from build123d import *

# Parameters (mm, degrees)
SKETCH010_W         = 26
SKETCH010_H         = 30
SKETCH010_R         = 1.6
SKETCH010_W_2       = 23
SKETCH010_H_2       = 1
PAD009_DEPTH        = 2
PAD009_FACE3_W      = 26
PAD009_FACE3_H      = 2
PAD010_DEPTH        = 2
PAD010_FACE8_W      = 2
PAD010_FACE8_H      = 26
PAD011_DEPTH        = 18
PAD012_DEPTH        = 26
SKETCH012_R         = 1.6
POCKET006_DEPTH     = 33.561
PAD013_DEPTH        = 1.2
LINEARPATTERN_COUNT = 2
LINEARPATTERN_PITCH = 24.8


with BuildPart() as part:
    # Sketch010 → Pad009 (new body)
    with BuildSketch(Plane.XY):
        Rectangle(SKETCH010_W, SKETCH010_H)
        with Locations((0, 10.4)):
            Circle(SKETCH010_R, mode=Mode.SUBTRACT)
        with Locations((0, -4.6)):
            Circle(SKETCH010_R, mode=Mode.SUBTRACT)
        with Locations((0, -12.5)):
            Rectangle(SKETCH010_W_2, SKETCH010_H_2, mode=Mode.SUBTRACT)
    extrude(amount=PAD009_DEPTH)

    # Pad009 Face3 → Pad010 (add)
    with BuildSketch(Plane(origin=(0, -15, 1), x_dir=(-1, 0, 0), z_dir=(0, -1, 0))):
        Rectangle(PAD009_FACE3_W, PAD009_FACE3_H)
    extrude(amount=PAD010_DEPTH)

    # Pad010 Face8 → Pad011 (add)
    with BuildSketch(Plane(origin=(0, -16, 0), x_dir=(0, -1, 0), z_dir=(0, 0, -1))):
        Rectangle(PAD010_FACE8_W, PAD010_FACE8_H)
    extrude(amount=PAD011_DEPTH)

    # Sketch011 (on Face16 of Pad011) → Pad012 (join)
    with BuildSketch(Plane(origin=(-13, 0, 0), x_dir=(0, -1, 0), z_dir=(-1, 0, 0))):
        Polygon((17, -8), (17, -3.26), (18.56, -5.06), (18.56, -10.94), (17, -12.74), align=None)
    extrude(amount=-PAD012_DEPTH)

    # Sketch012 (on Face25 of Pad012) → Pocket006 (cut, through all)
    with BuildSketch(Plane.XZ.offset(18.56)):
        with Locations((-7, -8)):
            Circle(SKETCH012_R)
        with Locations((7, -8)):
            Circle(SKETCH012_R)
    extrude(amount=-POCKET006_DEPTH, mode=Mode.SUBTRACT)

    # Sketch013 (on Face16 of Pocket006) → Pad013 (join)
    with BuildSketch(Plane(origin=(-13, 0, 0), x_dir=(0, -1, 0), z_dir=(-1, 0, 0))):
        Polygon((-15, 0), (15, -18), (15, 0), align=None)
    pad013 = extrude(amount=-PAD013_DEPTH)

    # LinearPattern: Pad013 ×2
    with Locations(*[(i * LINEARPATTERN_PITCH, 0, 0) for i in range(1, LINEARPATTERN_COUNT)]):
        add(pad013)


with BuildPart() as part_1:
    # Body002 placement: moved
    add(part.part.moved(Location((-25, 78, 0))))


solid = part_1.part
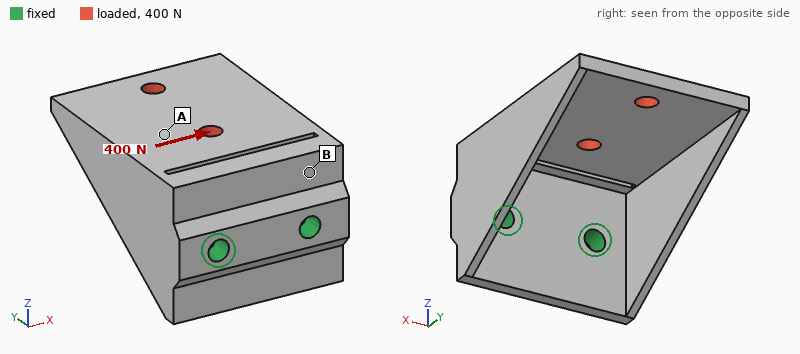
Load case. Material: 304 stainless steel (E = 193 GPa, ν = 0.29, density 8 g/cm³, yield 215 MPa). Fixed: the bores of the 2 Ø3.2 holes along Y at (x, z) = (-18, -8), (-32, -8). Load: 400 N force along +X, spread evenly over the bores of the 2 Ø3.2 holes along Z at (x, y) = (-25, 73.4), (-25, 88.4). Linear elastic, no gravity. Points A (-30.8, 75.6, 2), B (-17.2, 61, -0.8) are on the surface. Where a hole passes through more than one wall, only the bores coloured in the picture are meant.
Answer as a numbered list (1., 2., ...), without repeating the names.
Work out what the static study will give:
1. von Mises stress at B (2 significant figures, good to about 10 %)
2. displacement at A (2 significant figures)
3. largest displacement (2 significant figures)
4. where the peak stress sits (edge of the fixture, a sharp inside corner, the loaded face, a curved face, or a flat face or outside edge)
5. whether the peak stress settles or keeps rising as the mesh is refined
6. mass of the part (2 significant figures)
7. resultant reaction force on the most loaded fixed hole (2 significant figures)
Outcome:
1. 38 MPa
2. 23 µm
3. 54 µm
4. a sharp inside corner
5. keeps rising
6. 27 g
7. 460 N
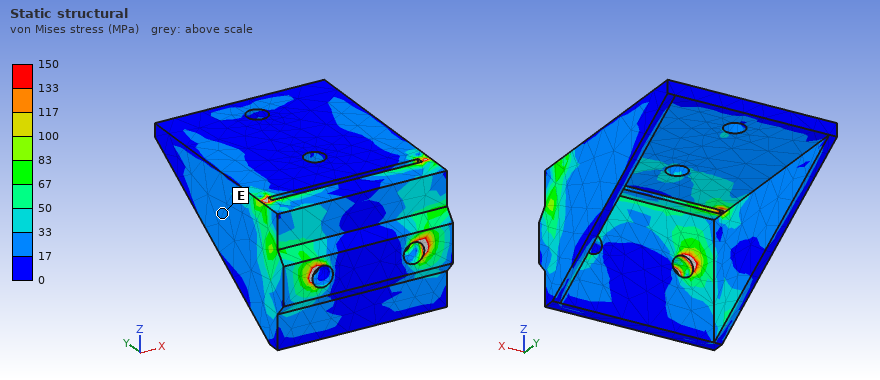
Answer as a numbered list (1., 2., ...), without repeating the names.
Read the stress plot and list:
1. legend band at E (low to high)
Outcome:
1. 17 to 33 MPa
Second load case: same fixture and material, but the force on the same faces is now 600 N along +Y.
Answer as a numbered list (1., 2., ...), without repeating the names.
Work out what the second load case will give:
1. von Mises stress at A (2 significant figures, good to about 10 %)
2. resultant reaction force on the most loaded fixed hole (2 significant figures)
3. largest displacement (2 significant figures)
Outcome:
1. 15 MPa
2. 310 N
3. 45 µm
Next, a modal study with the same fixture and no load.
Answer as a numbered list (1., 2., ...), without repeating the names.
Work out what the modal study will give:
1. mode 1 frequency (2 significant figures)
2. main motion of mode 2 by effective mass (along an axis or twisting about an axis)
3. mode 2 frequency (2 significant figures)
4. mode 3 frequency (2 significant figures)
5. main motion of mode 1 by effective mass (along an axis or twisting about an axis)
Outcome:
1. 3700 Hz
2. along X
3. 4200 Hz
4. 9600 Hz
5. along Z
